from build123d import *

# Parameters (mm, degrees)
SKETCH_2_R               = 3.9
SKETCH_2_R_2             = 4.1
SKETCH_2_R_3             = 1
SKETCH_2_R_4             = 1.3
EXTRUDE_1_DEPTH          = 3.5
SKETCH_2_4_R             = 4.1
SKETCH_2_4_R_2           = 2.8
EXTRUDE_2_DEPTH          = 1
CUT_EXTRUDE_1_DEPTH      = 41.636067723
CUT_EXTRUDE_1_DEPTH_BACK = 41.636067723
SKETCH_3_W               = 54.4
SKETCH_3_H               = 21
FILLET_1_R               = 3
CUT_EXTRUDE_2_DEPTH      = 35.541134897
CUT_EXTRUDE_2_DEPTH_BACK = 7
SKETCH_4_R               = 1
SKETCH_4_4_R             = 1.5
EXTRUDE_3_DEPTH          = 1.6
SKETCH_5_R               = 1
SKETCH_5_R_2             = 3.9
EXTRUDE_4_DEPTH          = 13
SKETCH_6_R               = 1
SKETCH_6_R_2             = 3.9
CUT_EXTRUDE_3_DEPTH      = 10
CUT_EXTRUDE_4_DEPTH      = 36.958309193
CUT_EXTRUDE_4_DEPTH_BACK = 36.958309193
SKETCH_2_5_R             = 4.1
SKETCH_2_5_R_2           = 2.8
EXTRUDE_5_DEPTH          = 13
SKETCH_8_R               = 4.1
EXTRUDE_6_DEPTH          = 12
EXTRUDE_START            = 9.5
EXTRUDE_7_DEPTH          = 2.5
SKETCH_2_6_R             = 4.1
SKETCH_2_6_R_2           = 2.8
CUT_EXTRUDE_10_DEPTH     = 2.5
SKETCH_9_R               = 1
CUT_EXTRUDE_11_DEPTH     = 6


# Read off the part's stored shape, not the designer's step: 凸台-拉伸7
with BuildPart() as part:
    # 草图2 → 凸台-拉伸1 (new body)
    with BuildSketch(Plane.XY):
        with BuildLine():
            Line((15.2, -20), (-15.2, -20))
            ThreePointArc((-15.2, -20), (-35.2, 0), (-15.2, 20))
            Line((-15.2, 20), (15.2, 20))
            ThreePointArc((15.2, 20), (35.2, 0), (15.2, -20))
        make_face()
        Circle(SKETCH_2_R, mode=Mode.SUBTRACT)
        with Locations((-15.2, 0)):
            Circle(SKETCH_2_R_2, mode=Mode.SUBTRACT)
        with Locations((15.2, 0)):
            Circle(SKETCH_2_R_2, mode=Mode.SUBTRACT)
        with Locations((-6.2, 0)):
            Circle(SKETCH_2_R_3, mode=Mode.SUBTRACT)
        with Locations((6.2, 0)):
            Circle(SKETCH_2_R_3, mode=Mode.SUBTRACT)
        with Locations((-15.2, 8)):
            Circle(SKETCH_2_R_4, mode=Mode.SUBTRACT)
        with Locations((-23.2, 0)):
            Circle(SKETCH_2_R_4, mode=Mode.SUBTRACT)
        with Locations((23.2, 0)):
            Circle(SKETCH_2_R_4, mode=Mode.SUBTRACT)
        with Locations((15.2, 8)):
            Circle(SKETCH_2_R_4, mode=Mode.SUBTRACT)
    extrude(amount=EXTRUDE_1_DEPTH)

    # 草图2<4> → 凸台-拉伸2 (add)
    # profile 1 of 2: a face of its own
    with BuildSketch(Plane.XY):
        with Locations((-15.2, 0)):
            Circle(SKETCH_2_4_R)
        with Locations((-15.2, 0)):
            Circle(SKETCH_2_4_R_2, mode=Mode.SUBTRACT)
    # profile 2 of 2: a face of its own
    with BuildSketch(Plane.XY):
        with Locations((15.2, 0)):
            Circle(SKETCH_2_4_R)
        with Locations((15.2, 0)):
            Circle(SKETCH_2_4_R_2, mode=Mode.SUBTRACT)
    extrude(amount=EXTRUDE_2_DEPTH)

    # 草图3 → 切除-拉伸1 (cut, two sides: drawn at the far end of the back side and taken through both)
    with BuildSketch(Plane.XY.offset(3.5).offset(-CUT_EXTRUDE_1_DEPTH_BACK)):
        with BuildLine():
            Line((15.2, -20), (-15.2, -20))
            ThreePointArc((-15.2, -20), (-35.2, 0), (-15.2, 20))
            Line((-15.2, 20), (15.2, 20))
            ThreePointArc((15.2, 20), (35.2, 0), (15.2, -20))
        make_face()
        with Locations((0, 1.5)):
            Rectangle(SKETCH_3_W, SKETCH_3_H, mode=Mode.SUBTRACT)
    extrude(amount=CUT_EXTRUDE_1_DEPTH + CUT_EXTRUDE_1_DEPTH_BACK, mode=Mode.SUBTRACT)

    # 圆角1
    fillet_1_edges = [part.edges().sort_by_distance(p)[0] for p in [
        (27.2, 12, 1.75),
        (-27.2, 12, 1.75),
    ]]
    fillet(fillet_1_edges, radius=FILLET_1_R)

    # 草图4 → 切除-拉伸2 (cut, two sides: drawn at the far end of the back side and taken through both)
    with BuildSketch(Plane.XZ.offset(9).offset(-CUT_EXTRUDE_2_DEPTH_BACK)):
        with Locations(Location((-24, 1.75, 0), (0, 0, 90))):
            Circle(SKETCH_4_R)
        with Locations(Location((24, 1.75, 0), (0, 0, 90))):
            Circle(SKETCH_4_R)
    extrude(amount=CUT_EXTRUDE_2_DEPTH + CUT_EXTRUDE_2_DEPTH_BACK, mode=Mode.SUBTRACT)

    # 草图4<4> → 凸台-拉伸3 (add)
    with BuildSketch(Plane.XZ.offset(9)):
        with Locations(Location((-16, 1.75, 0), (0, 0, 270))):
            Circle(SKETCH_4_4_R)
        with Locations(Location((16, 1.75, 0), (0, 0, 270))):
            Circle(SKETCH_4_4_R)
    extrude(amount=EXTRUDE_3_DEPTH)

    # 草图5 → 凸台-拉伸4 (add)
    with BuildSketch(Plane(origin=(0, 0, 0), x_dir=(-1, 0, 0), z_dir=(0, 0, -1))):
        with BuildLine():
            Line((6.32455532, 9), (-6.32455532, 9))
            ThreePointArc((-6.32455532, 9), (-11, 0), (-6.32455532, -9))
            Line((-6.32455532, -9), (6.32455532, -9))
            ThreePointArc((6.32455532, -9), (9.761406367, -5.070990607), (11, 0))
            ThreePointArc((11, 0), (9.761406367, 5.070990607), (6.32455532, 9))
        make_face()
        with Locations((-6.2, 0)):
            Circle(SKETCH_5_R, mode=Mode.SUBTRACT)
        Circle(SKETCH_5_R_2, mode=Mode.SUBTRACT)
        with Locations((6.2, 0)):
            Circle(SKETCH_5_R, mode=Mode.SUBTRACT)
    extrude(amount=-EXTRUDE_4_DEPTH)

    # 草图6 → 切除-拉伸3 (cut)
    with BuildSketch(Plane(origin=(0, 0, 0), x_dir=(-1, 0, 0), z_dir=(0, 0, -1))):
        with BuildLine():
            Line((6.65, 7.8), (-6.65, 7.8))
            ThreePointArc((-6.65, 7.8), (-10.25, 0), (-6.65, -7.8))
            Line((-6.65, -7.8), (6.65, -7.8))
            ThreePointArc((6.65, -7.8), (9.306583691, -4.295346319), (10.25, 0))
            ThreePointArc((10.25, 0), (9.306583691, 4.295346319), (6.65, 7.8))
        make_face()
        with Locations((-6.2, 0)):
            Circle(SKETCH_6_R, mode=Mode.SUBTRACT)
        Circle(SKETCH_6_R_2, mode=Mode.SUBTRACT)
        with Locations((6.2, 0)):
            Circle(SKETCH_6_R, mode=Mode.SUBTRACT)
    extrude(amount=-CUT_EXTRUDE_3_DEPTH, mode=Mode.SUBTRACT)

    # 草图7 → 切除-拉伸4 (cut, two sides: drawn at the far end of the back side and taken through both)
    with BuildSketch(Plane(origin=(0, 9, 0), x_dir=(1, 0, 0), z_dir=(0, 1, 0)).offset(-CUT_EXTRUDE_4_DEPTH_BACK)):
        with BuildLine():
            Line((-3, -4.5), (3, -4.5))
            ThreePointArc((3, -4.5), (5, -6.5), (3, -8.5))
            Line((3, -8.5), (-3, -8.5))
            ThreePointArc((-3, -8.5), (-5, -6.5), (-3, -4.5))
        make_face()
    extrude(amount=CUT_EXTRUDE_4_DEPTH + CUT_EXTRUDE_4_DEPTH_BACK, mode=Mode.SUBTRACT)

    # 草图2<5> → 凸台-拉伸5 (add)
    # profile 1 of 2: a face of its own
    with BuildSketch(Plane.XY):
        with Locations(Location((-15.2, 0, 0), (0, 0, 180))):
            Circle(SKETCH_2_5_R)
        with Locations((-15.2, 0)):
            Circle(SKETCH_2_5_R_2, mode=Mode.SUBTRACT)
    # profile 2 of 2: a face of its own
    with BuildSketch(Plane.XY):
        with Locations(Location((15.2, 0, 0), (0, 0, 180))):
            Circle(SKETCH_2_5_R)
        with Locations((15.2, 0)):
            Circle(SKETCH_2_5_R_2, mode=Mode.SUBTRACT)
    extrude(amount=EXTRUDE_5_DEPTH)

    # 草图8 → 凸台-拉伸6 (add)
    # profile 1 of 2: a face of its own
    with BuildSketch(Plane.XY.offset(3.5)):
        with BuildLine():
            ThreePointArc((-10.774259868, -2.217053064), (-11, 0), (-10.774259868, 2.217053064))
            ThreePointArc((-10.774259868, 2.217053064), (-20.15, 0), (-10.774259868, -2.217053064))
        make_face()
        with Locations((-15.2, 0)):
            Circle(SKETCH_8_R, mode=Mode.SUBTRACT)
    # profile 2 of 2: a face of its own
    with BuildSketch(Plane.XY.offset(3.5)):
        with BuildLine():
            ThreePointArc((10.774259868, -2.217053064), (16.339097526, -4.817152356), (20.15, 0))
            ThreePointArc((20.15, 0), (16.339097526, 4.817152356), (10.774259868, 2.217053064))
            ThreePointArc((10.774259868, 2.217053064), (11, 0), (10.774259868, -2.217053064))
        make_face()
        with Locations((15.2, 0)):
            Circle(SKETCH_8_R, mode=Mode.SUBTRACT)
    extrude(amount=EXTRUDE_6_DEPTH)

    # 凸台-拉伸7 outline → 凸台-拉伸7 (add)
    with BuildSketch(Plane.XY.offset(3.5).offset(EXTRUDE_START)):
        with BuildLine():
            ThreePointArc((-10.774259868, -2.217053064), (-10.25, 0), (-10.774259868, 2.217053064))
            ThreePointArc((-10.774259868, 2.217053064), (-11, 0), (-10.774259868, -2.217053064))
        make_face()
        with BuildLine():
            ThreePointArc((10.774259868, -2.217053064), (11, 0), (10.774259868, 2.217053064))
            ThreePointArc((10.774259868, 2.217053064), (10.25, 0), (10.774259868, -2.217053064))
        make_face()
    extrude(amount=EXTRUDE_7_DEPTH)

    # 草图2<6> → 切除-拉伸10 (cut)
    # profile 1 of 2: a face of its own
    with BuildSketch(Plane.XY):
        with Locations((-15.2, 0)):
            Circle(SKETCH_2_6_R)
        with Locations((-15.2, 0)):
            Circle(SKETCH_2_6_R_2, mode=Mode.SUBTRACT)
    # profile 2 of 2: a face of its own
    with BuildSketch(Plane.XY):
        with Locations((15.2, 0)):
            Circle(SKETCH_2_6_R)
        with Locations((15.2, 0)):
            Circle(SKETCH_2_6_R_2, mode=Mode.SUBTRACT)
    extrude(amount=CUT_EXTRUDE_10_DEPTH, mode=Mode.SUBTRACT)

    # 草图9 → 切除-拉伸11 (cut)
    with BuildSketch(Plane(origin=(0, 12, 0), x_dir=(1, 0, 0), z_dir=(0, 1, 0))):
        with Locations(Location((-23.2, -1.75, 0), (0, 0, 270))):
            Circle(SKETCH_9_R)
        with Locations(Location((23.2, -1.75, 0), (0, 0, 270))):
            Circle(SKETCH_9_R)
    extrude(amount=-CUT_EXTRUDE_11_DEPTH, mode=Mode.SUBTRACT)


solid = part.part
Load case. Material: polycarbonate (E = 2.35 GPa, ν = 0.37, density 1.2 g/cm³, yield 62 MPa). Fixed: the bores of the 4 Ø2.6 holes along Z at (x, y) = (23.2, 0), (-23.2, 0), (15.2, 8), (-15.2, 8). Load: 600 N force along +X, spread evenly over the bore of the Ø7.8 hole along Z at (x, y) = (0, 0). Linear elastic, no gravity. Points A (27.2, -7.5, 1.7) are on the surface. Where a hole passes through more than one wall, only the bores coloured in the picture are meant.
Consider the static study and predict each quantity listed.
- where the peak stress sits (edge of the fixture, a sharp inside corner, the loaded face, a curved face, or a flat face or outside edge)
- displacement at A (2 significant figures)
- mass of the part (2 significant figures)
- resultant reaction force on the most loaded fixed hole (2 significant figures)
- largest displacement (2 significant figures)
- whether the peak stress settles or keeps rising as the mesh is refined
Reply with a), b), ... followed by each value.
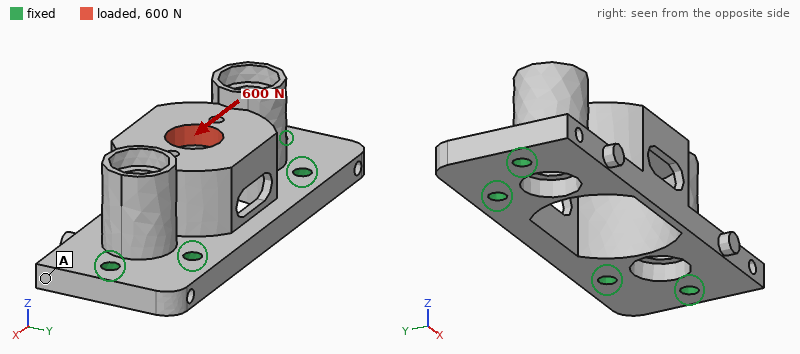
a) a sharp inside corner
b) 0.041 mm
c) 5.7 g
d) 230 N
e) 0.22 mm
f) keeps rising
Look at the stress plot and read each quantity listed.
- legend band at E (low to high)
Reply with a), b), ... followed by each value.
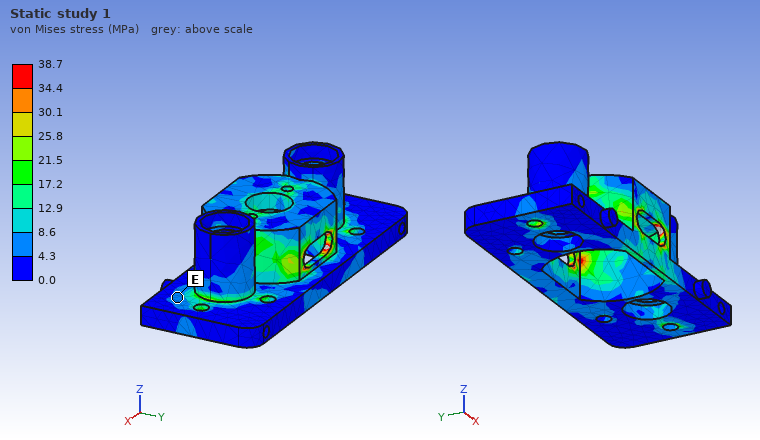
a) 4.3 to 8.6 MPa
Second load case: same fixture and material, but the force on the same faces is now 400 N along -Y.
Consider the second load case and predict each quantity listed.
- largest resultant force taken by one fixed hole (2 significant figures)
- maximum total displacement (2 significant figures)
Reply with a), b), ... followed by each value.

a) 250 N
b) 0.71 mm
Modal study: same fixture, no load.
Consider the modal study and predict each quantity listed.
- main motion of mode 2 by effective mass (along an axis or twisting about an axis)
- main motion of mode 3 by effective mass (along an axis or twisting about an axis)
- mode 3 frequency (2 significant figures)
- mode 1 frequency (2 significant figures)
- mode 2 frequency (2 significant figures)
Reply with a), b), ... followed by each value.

a) along X
b) along Z
c) 6000 Hz
d) 2700 Hz
e) 5400 Hz
